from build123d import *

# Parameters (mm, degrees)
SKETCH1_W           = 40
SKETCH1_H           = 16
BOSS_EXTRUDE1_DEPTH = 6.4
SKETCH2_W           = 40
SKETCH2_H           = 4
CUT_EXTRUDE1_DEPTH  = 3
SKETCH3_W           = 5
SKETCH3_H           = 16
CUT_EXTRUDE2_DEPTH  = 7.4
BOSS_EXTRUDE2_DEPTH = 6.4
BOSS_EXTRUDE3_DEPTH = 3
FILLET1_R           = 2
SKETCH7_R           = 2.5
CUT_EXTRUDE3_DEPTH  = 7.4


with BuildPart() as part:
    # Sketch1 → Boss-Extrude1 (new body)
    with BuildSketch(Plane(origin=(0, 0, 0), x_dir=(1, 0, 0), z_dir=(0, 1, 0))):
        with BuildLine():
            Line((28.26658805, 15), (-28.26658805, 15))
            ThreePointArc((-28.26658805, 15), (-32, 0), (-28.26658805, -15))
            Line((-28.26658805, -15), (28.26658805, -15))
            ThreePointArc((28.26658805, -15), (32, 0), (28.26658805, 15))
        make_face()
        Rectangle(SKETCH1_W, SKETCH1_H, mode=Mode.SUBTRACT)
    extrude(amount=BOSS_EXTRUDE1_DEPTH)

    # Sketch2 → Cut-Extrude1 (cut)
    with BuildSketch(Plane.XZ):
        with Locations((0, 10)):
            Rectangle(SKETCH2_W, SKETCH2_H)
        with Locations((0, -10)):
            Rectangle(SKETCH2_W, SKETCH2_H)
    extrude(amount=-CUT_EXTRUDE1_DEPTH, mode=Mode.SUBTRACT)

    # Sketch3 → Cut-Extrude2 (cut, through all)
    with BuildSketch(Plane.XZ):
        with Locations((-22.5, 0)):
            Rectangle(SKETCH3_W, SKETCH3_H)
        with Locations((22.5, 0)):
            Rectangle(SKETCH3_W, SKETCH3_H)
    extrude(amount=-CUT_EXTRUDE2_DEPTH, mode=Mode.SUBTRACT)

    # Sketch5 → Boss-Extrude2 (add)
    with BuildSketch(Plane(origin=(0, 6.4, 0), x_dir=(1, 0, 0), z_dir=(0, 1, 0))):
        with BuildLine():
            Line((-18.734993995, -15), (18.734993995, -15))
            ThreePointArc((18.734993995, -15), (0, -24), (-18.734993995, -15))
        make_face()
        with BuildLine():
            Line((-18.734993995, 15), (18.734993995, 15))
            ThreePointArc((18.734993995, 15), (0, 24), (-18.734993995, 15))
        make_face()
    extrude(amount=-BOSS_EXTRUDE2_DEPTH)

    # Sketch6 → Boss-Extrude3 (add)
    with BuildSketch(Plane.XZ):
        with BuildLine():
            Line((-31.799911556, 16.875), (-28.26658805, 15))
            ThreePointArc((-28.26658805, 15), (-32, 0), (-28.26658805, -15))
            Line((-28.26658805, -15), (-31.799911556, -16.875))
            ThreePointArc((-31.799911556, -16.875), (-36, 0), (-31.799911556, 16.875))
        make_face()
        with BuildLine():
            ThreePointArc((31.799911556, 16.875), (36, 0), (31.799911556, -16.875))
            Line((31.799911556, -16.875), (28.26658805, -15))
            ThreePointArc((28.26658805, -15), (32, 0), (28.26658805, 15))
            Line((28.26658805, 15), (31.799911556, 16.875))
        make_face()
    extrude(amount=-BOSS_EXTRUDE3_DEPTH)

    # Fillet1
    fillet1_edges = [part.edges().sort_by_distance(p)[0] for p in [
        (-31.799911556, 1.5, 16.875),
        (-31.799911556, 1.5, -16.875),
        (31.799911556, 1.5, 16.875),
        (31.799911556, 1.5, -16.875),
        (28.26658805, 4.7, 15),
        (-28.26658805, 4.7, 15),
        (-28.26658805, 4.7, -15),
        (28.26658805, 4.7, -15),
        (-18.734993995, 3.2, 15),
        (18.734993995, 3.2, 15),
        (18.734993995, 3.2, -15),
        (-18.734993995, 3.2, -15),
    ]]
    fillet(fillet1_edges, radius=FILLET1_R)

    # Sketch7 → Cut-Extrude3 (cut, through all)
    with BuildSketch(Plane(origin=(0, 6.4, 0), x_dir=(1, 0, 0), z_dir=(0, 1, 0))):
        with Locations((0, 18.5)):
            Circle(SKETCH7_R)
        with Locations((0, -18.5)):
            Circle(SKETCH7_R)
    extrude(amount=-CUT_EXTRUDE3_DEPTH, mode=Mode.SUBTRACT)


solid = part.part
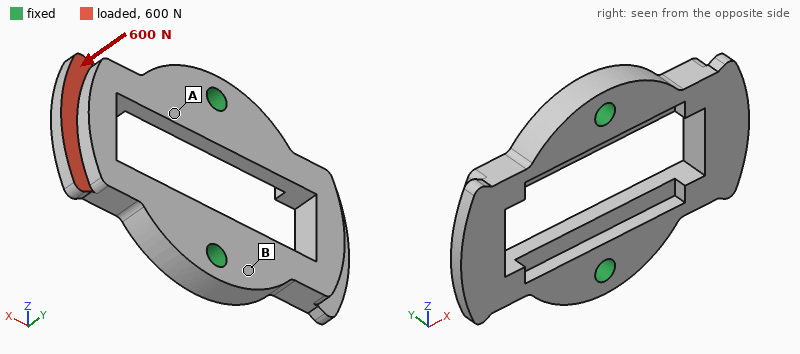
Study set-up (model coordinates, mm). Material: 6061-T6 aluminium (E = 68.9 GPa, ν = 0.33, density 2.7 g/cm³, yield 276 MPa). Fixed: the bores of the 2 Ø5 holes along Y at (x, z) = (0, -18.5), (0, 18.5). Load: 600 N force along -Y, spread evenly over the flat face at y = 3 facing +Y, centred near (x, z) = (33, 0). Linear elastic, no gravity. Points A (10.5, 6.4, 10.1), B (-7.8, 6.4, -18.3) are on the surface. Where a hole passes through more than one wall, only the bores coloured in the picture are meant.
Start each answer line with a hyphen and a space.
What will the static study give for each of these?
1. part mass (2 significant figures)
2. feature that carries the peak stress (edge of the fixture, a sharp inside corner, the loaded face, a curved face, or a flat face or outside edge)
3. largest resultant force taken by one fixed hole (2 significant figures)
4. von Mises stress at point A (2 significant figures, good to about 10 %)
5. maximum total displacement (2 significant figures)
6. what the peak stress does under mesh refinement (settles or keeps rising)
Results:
- 25 g
- edge of the fixture
- 330 N
- 86 MPa
- 0.31 mm
- keeps rising
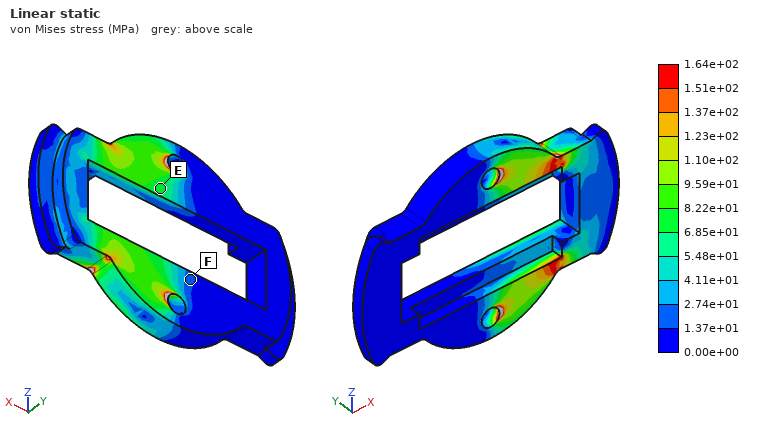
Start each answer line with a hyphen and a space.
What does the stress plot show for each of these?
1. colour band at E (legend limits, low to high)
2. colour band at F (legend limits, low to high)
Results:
- 6.85e+01 to 8.22e+01 MPa
- 1.37e+01 to 2.74e+01 MPa
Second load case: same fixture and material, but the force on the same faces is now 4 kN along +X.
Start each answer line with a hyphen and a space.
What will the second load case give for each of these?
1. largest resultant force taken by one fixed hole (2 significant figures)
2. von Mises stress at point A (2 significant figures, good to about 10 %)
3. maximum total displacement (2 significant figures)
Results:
- 2.1 kN
- 20 MPa
- 51 µm
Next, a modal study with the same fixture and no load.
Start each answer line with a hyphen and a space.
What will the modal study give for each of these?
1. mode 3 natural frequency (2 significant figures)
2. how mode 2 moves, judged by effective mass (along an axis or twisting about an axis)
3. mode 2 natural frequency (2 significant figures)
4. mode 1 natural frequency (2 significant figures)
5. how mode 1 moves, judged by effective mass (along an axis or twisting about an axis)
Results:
- 9600 Hz
- along Y
- 4300 Hz
- 4100 Hz
- twisting about Z
